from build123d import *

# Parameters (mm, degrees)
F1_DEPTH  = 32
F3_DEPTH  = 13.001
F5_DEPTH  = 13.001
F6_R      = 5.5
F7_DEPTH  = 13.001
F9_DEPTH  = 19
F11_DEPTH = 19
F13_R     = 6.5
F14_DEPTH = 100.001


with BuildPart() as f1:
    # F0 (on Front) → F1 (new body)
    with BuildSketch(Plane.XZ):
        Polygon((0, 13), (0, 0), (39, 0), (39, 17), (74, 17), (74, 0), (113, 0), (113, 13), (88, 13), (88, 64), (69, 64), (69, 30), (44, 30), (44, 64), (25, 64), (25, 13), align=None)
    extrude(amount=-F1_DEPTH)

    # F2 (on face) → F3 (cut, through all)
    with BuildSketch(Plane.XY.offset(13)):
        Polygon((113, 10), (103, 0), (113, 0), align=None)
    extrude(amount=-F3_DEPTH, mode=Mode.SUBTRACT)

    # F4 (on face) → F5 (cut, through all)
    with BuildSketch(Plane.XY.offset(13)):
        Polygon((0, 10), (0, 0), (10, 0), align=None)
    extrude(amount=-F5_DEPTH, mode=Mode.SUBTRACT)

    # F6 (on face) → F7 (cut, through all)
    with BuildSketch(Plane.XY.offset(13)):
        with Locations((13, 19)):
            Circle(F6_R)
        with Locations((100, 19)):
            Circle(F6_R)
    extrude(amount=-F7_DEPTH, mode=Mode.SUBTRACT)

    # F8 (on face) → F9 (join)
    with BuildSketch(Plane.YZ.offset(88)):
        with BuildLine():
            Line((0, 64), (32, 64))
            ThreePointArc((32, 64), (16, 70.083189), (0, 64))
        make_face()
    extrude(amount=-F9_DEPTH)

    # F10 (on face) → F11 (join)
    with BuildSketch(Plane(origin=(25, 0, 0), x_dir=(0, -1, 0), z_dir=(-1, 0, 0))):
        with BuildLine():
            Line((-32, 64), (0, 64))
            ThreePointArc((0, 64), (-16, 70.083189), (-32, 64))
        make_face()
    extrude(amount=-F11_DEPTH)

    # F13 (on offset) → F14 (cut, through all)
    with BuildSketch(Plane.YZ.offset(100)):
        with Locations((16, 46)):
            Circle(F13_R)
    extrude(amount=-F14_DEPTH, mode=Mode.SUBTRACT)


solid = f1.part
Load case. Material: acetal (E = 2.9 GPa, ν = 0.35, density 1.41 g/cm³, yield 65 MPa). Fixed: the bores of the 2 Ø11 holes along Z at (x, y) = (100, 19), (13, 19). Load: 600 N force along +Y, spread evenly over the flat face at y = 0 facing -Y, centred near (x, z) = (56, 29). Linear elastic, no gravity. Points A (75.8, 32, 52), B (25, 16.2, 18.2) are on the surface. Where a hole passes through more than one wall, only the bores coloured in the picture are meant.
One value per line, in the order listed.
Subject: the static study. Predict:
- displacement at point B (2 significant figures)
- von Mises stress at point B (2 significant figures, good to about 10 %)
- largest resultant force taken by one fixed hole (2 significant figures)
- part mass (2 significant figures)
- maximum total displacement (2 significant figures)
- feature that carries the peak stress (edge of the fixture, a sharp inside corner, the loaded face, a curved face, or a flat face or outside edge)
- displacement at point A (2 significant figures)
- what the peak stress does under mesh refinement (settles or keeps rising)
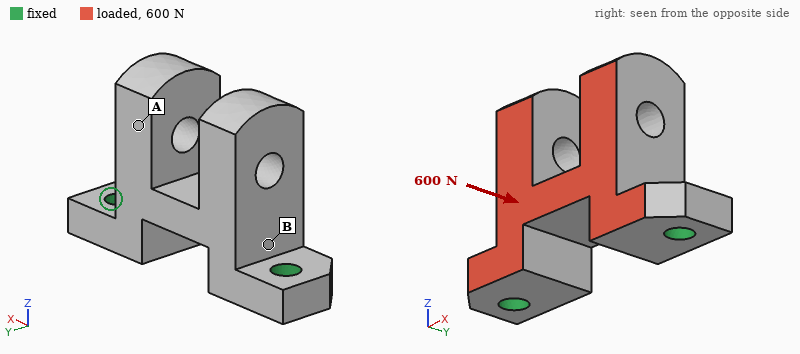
0.069 mm
2.6 MPa
300 N
140 g
0.34 mm
edge of the fixture
0.26 mm
keeps rising
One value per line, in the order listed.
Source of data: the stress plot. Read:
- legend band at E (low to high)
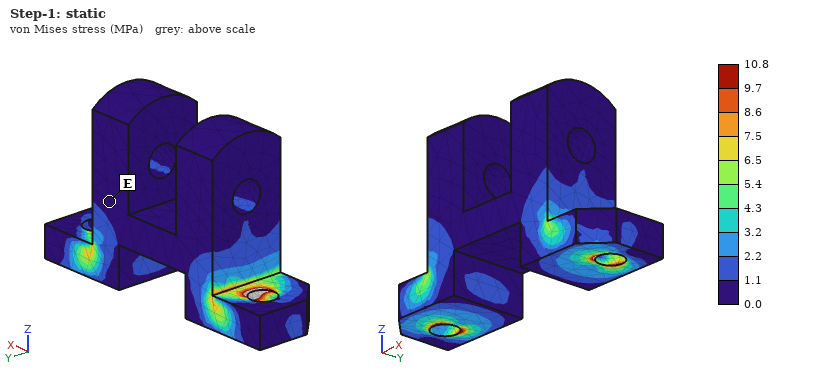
0.0 to 1.1 MPa
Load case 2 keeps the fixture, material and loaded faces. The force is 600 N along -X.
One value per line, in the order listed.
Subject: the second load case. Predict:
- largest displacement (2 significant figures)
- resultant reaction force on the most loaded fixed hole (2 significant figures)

0.11 mm
360 N
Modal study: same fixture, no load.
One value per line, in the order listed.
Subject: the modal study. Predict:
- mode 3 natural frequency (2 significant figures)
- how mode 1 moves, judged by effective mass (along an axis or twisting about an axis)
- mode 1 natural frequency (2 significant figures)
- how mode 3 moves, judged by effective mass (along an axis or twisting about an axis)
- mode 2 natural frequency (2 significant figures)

1300 Hz
along Y
690 Hz
along X
1100 Hz
